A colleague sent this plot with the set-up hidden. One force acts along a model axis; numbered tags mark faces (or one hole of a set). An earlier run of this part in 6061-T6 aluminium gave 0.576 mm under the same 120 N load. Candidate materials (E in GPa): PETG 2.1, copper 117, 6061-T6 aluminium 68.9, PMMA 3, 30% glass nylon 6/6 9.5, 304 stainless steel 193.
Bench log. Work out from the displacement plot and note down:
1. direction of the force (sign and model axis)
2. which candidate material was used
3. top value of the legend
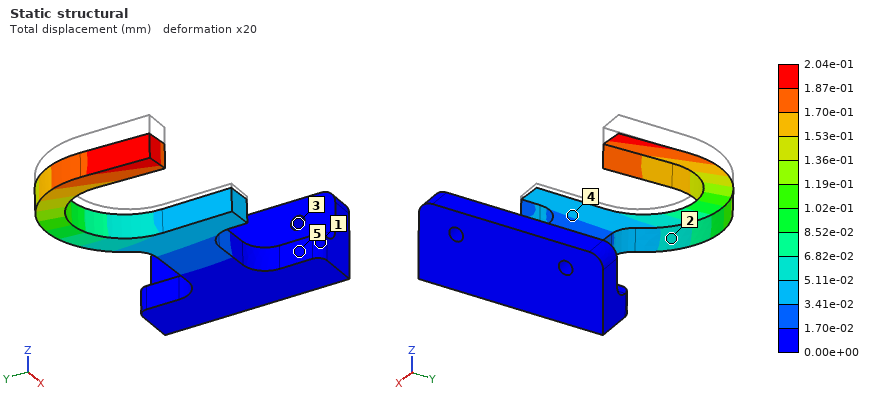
-Z
304 stainless steel
2.04e-01 mm
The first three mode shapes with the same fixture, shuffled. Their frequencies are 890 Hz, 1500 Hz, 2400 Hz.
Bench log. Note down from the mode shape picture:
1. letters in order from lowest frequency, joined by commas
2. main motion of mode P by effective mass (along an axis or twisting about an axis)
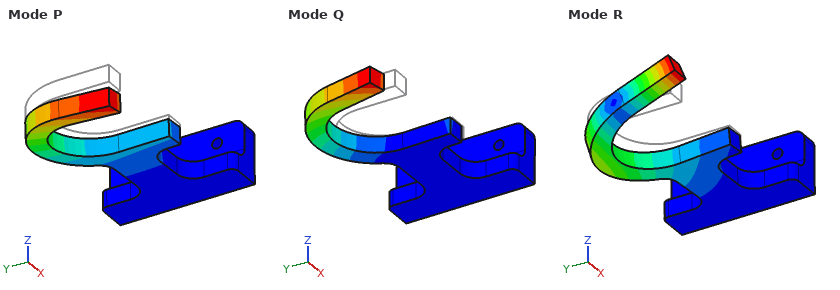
P, Q, R
along Z
